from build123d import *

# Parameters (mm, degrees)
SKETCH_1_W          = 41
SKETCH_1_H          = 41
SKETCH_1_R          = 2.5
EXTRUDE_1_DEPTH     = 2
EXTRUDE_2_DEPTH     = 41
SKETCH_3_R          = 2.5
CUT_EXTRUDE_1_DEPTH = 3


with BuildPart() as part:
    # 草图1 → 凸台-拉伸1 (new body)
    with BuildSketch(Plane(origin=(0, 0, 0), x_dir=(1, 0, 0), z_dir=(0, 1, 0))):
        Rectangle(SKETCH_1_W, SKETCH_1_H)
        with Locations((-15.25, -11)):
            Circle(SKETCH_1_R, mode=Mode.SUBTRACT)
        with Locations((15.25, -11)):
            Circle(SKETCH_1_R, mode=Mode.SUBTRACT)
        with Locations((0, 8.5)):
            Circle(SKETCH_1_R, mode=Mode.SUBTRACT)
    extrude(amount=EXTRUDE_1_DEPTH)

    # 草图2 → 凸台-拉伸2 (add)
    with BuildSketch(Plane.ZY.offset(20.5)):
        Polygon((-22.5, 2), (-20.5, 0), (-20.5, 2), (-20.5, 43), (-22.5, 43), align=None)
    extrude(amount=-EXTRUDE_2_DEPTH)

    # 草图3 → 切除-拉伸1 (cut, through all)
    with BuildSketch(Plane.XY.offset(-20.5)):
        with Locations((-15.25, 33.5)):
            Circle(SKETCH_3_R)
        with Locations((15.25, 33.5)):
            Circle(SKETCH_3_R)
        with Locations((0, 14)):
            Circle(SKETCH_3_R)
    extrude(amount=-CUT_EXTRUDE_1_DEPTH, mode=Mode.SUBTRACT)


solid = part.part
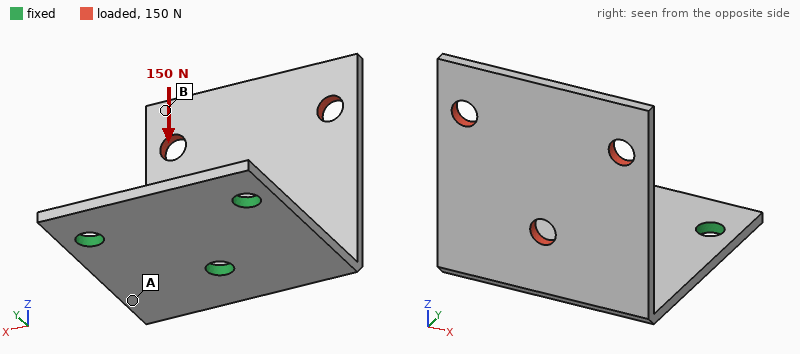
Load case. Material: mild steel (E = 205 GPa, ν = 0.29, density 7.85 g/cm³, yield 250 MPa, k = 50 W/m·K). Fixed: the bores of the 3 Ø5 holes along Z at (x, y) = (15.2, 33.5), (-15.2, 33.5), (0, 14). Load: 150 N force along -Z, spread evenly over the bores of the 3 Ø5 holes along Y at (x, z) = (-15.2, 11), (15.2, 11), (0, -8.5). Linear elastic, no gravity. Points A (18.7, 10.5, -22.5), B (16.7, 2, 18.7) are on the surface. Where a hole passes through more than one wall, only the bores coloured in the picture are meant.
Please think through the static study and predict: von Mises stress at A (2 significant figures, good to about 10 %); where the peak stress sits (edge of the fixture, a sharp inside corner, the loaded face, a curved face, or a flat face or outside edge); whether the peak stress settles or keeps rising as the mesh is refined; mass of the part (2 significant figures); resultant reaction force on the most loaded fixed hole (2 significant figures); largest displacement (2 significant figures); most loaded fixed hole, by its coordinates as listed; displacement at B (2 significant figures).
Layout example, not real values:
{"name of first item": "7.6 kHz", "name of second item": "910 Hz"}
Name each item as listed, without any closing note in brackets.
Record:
{"von Mises stress at A": "23 MPa", "where the peak stress sits": "edge of the fixture", "whether the peak stress settles or keeps rising as the mesh is refined": "keeps rising", "mass of the part": "52 g", "resultant reaction force on the most loaded fixed hole": "180 N", "largest displacement": "0.10 mm", "most loaded fixed hole, by its coordinates as listed": "(0, 14)", "displacement at B": "0.096 mm"}
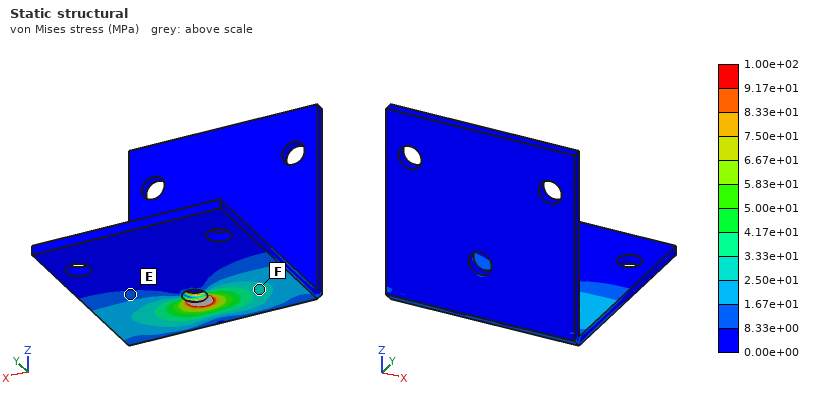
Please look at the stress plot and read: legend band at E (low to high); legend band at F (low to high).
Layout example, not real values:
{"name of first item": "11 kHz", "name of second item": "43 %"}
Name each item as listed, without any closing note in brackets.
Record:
{"legend band at E": "8.33e+00 to 1.67e+01 MPa", "legend band at F": "2.50e+01 to 3.33e+01 MPa"}
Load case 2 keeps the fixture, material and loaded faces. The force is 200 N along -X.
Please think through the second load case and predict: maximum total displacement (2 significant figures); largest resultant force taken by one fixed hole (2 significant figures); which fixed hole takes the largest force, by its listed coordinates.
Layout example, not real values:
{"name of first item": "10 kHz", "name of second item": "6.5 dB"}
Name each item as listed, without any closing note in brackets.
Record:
{"maximum total displacement": "0.30 mm", "largest resultant force taken by one fixed hole": "210 N", "which fixed hole takes the largest force, by its listed coordinates": "(0, 14)"}
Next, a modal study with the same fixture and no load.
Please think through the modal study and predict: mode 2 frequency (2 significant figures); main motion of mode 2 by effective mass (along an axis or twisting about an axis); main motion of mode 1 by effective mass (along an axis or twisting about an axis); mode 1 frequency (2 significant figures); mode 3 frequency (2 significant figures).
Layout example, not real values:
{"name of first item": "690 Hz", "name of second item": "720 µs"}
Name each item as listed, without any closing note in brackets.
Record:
{"mode 2 frequency": "1000 Hz", "main motion of mode 2 by effective mass": "along X", "main motion of mode 1 by effective mass": "along Y", "mode 1 frequency": "630 Hz", "mode 3 frequency": "2200 Hz"}
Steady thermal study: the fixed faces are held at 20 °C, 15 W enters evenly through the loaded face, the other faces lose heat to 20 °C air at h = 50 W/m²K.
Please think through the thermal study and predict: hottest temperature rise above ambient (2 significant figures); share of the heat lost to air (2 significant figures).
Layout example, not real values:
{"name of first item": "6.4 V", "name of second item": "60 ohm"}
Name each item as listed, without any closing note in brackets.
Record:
{"hottest temperature rise above ambient": "78 K", "share of the heat lost to air": "67 %"}
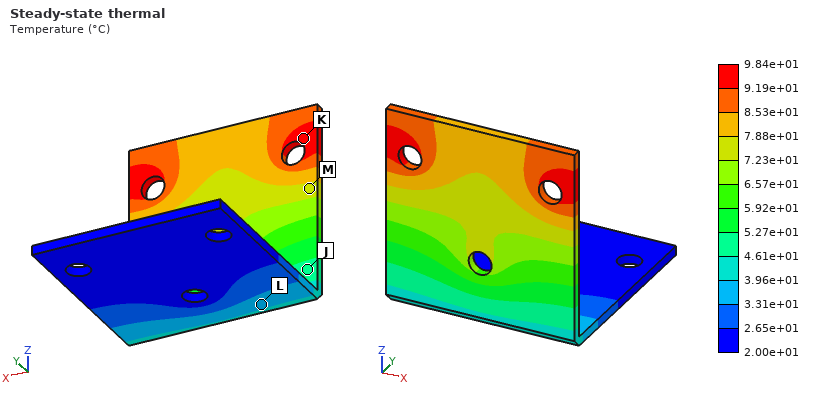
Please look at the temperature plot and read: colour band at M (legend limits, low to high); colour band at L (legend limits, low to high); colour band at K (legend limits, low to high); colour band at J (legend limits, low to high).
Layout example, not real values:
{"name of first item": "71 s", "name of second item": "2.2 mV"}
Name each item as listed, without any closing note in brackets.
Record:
{"colour band at M": "7.23e+01 to 7.88e+01 °C", "colour band at L": "3.31e+01 to 3.96e+01 °C", "colour band at K": "9.19e+01 to 9.84e+01 °C", "colour band at J": "4.61e+01 to 5.27e+01 °C"}
